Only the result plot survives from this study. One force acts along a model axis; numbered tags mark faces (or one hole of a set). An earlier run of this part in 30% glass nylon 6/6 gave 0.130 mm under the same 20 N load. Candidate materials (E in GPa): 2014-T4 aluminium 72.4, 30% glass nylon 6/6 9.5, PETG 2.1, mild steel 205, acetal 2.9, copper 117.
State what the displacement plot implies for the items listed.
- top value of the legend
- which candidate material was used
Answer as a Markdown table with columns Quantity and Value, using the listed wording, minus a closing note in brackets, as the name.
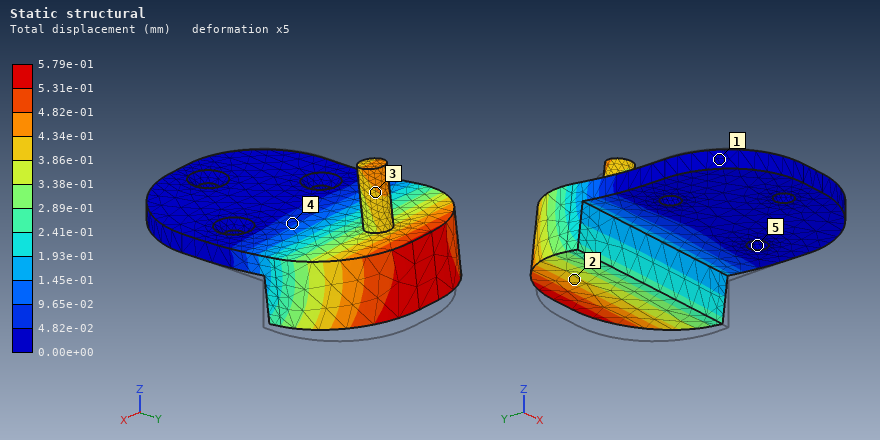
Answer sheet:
| Quantity | Value |
|---|---|
| top value of the legend | 5.79e-01 mm |
| which candidate material was used | PETG |
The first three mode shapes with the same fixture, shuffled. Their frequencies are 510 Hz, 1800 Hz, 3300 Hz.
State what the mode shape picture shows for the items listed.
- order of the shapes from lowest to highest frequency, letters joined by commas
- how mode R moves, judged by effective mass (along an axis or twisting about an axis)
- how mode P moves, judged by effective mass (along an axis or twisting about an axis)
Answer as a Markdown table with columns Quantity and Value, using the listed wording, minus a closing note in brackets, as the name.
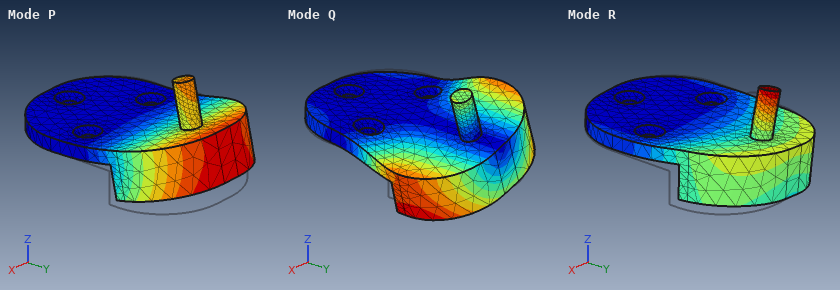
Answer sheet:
| Quantity | Value |
|---|---|
| order of the shapes from lowest to highest frequency, letters joined by commas | P, Q, R |
| how mode R moves, judged by effective mass | along X |
| how mode P moves, judged by effective mass | along Z |
